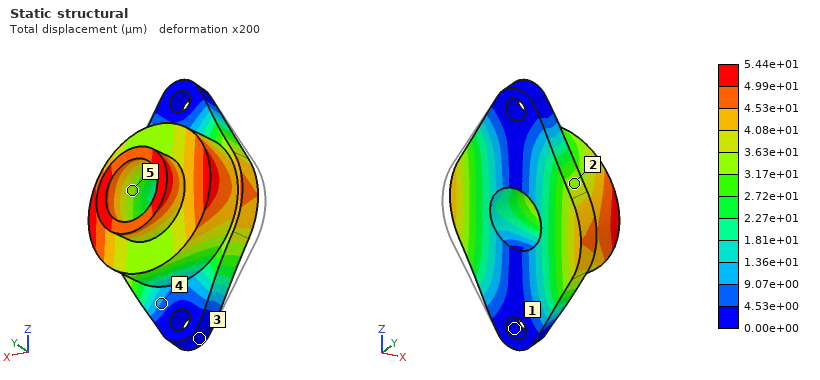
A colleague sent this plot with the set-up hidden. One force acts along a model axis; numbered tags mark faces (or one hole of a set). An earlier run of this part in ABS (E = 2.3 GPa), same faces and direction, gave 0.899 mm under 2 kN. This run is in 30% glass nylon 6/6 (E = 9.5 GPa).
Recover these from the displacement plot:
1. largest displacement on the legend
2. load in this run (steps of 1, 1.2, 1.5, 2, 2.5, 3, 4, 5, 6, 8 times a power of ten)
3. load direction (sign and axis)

5.44e+01 µm
500 N
+X
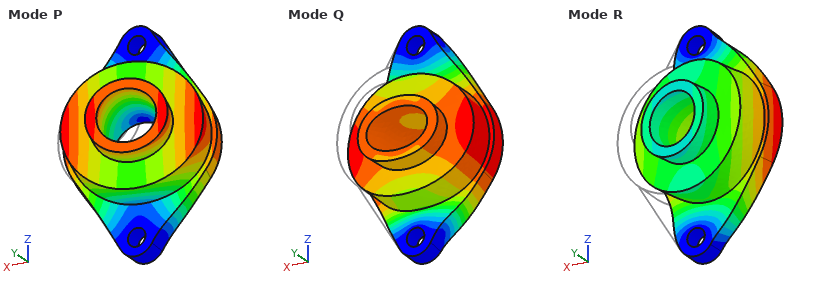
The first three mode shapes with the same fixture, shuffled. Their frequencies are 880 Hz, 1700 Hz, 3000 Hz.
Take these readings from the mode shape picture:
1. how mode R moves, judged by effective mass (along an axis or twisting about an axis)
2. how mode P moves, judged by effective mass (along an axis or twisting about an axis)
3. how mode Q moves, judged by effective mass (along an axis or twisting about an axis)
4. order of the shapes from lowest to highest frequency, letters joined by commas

along X
along X
along Y
P, Q, R
